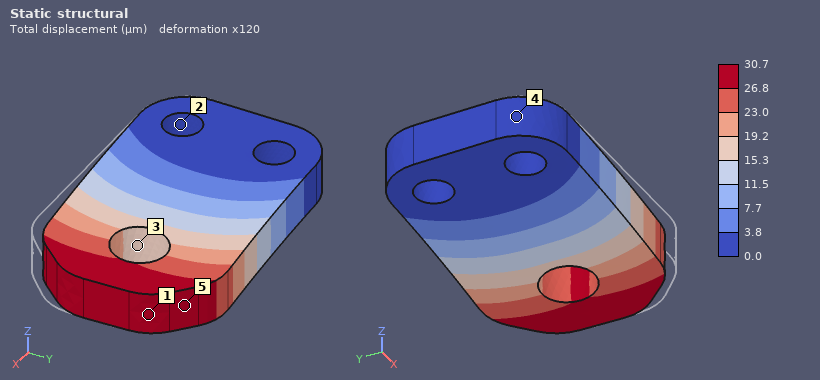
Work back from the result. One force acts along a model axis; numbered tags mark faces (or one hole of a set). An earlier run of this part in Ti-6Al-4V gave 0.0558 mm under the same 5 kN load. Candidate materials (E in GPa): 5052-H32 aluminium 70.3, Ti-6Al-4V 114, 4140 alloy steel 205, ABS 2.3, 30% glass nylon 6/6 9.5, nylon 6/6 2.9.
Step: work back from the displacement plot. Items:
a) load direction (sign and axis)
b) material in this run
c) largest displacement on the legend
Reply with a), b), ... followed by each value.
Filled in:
a) +Y
b) 4140 alloy steel
c) 30.7 µm
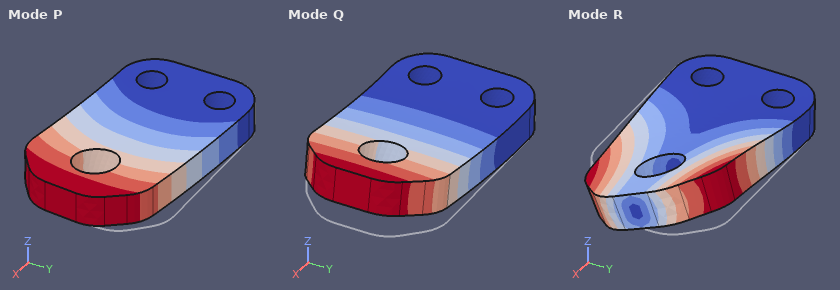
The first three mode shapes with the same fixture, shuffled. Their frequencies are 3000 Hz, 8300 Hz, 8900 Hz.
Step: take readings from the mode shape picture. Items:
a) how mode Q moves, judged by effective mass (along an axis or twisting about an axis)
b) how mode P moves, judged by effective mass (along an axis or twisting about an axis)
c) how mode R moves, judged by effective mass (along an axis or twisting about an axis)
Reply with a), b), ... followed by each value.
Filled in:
a) along Z
b) along Y
c) twisting about X
